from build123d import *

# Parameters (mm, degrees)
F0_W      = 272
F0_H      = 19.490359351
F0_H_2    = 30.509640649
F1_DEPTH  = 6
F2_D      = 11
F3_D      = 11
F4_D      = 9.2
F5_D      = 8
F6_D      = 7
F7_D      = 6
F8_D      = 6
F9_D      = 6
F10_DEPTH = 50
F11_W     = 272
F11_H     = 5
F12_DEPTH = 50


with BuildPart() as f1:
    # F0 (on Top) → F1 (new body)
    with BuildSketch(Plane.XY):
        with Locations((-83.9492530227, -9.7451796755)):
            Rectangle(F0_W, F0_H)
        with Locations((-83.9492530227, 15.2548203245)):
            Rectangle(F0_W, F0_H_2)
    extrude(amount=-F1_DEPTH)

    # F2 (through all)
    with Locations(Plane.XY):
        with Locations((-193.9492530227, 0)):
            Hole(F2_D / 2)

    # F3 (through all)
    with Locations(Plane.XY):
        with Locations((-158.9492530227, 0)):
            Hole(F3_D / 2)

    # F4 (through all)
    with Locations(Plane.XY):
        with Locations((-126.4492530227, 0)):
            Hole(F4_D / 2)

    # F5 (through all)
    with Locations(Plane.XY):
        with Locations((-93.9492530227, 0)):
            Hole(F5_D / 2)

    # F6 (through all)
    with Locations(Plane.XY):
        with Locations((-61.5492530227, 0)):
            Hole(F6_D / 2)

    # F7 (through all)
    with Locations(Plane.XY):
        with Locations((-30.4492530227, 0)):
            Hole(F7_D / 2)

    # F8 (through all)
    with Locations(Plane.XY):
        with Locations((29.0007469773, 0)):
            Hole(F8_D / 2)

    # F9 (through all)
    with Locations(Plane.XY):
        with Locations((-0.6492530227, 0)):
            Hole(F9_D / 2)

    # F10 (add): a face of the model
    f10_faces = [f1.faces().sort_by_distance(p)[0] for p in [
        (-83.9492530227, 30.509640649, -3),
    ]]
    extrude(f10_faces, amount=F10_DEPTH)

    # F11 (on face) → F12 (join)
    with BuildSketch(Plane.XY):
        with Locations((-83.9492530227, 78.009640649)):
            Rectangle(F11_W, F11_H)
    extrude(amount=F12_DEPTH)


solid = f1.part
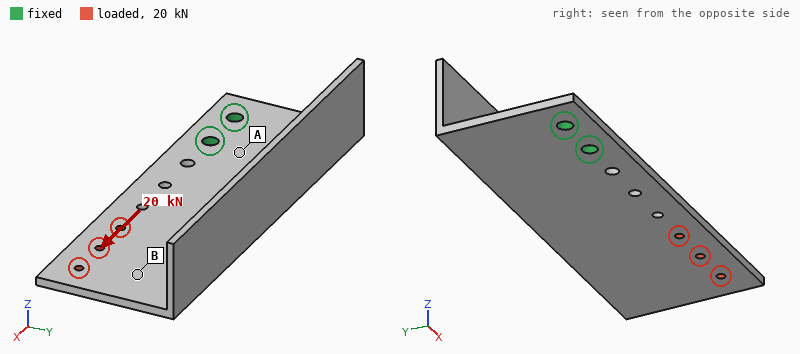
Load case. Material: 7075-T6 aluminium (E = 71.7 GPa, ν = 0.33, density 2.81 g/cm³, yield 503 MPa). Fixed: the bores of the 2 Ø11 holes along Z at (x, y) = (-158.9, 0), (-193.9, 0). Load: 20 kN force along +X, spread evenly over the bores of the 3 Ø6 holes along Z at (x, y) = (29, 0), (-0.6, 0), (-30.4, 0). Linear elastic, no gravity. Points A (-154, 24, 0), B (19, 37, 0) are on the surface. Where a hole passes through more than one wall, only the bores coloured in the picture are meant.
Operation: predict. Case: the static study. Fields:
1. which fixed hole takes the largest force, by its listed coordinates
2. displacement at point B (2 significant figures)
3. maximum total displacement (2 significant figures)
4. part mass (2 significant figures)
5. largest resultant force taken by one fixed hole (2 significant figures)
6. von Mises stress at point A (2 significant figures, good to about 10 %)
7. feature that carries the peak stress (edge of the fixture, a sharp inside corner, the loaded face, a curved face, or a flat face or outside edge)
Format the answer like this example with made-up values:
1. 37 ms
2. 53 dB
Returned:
1. (-158.9, 0)
2. 0.27 mm
3. 0.41 mm
4. 640 g
5. 16 kN
6. 28 MPa
7. a curved face
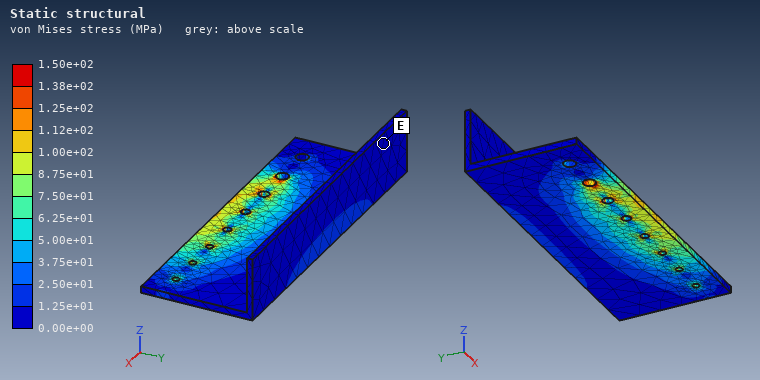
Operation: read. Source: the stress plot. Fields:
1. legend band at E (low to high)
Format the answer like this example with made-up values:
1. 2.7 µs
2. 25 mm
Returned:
1. 0.00e+00 to 1.25e+01 MPa
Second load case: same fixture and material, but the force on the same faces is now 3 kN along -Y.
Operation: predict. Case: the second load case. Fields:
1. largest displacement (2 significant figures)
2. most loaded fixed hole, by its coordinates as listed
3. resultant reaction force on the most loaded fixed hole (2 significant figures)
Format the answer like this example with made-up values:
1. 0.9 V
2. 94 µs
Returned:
1. 0.54 mm
2. (-158.9, 0)
3. 13 kN
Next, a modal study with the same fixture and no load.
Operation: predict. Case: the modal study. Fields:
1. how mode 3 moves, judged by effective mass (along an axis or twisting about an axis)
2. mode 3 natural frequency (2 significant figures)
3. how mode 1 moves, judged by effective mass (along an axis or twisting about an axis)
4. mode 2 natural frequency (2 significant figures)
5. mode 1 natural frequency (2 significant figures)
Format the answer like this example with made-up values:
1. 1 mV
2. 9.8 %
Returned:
1. along Z
2. 520 Hz
3. along Z
4. 280 Hz
5. 120 Hz
